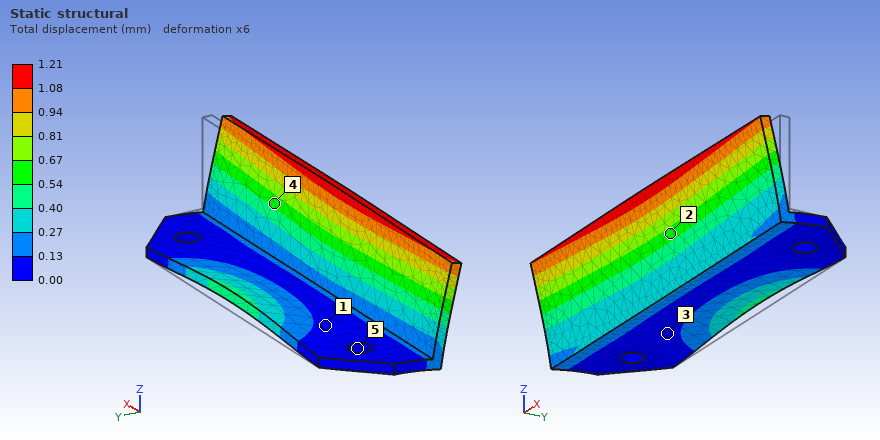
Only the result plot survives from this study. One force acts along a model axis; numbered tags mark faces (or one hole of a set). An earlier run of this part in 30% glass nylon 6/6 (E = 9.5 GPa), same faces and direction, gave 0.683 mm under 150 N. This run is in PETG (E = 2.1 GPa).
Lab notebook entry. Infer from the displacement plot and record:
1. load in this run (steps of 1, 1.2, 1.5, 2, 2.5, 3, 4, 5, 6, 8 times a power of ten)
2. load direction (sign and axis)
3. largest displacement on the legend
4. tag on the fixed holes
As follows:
60 N
-Y
1.21 mm
5
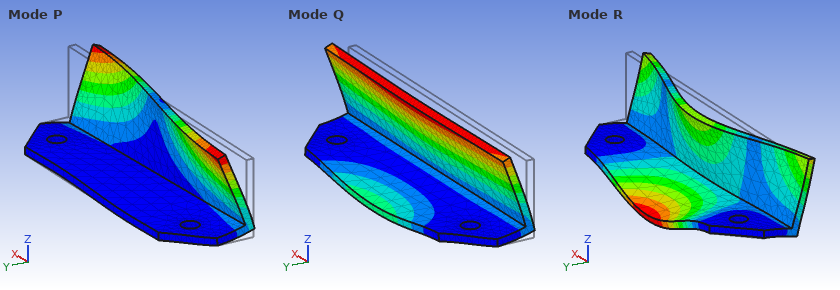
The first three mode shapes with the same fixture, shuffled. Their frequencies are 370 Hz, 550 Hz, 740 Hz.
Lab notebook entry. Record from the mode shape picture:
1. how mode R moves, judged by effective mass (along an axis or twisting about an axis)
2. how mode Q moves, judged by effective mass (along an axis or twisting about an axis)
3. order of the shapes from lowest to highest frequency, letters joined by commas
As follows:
along Z
along Y
Q, P, R
